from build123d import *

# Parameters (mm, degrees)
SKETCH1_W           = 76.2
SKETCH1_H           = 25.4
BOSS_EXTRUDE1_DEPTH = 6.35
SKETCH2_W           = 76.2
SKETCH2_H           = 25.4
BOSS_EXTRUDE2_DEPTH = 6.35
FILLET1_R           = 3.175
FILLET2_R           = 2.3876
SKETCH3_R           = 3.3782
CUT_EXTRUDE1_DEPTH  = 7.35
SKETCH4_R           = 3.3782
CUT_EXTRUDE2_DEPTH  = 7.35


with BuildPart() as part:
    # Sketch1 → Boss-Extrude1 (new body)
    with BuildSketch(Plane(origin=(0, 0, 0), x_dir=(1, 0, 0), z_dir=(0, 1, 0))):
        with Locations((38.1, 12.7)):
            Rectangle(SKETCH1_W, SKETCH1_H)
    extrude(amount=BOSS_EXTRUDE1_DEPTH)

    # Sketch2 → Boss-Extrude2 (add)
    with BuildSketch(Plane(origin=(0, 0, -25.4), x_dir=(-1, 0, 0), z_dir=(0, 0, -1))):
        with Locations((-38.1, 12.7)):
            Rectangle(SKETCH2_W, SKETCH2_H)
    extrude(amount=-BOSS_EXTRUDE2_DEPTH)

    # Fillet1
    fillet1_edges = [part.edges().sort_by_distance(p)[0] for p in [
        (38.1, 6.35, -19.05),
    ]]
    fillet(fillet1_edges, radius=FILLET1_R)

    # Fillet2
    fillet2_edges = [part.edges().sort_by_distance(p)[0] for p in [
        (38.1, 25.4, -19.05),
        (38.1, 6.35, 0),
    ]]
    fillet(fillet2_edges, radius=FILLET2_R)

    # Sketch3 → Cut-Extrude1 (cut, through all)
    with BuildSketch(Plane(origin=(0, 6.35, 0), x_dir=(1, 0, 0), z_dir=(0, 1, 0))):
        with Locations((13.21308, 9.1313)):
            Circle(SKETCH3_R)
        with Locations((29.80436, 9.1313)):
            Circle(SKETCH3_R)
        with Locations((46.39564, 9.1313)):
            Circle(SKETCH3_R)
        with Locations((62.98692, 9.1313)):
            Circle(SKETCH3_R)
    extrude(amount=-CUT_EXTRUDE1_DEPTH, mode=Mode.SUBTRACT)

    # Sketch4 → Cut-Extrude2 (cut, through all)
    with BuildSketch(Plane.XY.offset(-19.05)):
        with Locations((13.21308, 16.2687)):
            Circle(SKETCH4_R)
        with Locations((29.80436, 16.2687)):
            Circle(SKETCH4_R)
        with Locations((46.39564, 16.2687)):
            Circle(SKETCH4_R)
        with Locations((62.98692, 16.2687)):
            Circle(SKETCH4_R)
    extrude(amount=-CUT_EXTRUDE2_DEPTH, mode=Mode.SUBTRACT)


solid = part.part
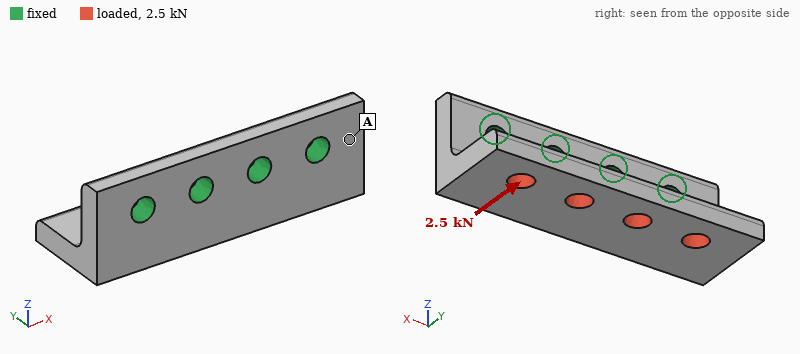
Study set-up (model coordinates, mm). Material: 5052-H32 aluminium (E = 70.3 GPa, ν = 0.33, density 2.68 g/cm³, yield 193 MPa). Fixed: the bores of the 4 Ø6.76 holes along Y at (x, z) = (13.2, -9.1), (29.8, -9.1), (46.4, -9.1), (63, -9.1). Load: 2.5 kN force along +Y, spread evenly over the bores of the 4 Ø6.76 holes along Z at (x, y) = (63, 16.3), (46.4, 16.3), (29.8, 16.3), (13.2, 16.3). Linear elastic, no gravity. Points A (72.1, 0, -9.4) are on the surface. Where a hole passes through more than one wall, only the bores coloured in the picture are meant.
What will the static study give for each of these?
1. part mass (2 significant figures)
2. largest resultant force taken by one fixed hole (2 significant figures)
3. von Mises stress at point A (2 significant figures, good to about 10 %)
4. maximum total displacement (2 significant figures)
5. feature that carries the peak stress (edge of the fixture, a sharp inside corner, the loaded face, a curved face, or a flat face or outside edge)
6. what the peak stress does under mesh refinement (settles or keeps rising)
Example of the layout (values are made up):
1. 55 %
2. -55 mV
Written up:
1. 53 g
2. 640 N
3. 16 MPa
4. 38 µm
5. edge of the fixture
6. keeps rising
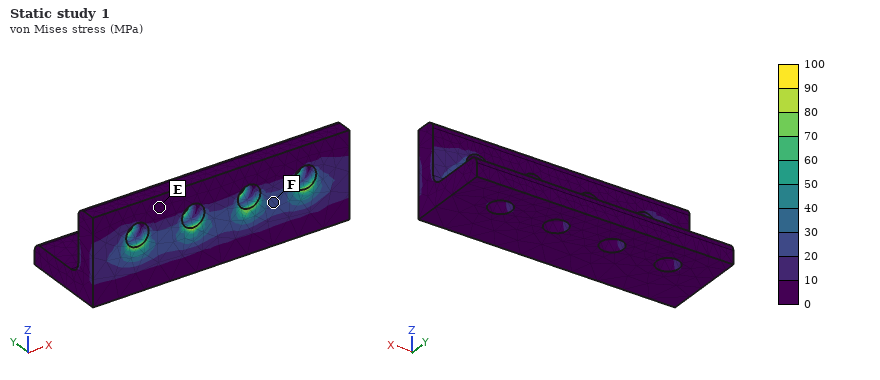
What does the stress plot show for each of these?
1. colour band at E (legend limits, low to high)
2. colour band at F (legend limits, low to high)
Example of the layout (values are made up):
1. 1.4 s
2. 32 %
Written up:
1. 0 to 10 MPa
2. 20 to 30 MPa
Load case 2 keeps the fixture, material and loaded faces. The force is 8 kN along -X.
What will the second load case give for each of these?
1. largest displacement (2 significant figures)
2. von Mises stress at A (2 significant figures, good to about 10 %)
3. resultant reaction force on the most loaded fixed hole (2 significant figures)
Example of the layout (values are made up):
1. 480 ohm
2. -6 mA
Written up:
1. 72 µm
2. 45 MPa
3. 3.0 kN
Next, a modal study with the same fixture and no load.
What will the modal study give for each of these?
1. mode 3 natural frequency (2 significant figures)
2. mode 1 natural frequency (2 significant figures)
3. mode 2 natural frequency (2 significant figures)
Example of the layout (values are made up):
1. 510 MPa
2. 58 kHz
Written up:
1. 15 kHz
2. 6600 Hz
3. 8100 Hz
